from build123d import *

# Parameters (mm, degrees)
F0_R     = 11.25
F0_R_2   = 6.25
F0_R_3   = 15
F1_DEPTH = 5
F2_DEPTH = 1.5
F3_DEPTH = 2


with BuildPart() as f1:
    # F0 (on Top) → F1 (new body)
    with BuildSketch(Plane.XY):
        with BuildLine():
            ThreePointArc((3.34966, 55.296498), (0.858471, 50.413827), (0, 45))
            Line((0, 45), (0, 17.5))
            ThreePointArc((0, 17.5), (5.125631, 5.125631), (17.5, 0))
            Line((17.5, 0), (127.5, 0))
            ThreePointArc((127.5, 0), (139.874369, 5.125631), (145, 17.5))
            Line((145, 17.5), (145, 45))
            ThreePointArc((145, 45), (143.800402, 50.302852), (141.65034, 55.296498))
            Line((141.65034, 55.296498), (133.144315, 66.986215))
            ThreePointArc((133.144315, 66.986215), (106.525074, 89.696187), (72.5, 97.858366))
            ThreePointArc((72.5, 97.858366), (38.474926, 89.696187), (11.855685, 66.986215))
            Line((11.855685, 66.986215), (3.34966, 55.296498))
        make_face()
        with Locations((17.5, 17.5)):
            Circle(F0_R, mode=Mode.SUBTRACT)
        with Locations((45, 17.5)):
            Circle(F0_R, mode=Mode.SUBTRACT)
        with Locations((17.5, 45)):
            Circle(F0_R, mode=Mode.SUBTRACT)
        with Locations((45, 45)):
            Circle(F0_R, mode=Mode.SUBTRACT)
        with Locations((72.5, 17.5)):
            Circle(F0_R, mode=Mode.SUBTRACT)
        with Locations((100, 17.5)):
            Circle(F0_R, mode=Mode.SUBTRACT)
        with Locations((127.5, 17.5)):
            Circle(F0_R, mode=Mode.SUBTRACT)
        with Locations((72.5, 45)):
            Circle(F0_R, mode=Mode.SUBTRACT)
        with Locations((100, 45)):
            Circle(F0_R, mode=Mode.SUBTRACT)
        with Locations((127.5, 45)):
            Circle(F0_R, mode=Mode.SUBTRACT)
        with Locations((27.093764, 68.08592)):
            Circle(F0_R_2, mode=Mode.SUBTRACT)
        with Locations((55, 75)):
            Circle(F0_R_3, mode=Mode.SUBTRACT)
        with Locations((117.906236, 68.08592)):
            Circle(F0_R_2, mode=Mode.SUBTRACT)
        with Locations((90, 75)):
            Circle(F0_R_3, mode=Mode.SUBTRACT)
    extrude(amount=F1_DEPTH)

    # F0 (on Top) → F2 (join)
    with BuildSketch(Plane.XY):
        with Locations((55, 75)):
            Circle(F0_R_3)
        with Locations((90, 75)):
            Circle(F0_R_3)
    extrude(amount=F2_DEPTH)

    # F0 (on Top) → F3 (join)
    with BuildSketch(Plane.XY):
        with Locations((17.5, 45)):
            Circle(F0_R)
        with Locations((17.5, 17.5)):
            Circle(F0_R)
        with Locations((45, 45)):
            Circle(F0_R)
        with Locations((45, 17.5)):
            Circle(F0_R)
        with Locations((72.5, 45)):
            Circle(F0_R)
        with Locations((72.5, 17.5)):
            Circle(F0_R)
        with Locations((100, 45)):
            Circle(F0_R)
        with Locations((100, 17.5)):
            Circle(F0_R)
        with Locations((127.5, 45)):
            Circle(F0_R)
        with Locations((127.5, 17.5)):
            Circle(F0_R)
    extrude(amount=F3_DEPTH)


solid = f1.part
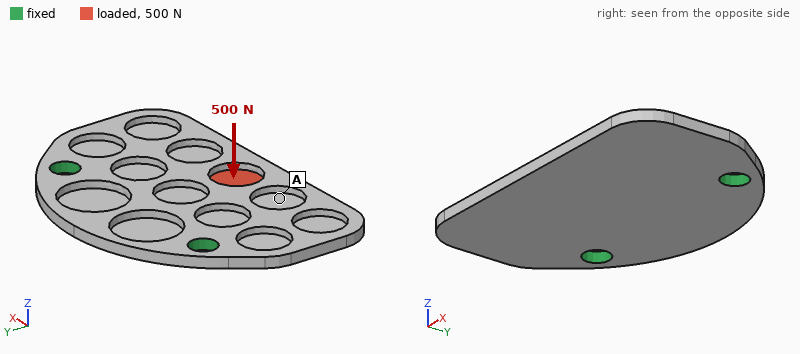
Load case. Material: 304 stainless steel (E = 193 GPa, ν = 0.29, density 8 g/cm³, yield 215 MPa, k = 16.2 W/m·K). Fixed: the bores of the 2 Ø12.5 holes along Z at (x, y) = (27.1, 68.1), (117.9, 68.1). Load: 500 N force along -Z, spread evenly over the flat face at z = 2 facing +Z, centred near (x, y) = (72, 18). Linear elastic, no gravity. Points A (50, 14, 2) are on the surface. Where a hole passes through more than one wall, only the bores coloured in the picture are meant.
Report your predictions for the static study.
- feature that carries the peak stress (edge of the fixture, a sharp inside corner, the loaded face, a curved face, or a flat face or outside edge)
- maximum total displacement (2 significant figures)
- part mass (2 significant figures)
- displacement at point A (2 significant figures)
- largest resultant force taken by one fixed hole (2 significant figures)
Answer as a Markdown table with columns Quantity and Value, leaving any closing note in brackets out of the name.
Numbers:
| Quantity | Value |
|---|---|
| feature that carries the peak stress | a curved face |
| maximum total displacement | 0.28 mm |
| part mass | 340 g |
| displacement at point A | 0.19 mm |
| largest resultant force taken by one fixed hole | 270 N |
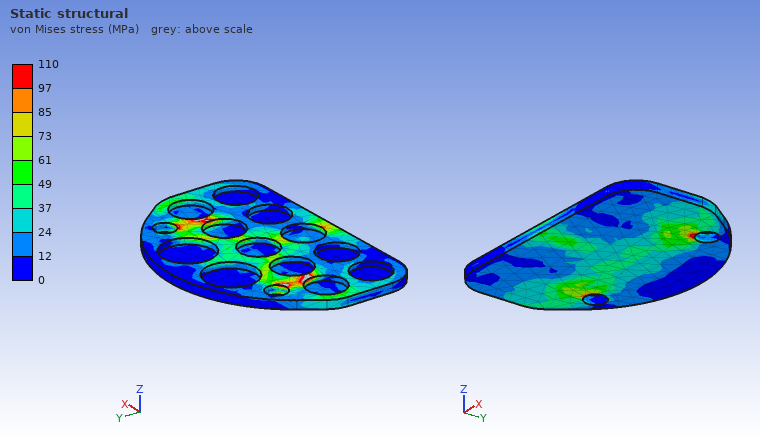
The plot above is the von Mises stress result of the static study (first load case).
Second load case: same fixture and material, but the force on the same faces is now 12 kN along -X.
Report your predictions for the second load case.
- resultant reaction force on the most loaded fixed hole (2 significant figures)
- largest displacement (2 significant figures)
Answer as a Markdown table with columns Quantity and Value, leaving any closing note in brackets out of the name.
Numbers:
| Quantity | Value |
|---|---|
| resultant reaction force on the most loaded fixed hole | 8.3 kN |
| largest displacement | 61 µm |
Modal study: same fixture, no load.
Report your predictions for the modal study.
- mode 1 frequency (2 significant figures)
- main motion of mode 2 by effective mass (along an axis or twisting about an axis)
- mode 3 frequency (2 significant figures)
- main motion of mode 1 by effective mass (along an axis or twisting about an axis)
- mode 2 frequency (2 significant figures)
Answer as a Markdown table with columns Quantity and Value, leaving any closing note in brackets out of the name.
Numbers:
| Quantity | Value |
|---|---|
| mode 1 frequency | 740 Hz |
| main motion of mode 2 by effective mass | twisting about Y |
| mode 3 frequency | 1900 Hz |
| main motion of mode 1 by effective mass | along Z |
| mode 2 frequency | 1100 Hz |
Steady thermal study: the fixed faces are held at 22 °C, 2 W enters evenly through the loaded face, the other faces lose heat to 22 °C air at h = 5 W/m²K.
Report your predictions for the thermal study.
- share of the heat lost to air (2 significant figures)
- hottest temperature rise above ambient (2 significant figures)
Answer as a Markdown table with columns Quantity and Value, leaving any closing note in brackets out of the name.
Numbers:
| Quantity | Value |
|---|---|
| share of the heat lost to air | 41 % |
| hottest temperature rise above ambient | 21 K |
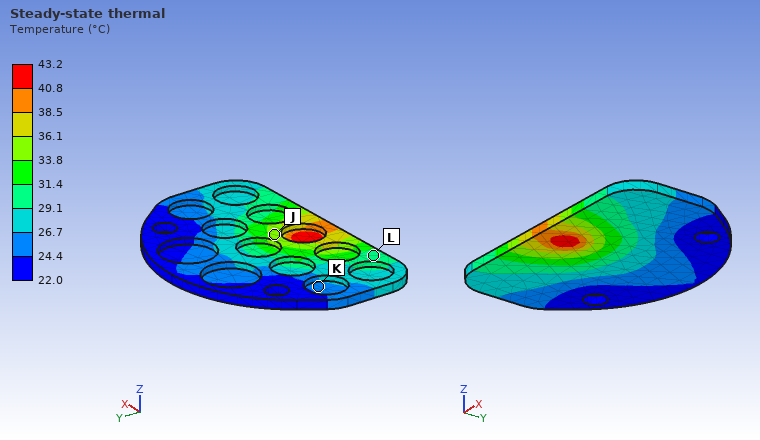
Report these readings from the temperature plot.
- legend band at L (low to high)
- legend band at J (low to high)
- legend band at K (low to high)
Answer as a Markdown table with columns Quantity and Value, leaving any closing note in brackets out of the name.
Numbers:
| Quantity | Value |
|---|---|
| legend band at L | 29.1 to 31.4 °C |
| legend band at J | 33.8 to 36.1 °C |
| legend band at K | 24.4 to 26.7 °C |
